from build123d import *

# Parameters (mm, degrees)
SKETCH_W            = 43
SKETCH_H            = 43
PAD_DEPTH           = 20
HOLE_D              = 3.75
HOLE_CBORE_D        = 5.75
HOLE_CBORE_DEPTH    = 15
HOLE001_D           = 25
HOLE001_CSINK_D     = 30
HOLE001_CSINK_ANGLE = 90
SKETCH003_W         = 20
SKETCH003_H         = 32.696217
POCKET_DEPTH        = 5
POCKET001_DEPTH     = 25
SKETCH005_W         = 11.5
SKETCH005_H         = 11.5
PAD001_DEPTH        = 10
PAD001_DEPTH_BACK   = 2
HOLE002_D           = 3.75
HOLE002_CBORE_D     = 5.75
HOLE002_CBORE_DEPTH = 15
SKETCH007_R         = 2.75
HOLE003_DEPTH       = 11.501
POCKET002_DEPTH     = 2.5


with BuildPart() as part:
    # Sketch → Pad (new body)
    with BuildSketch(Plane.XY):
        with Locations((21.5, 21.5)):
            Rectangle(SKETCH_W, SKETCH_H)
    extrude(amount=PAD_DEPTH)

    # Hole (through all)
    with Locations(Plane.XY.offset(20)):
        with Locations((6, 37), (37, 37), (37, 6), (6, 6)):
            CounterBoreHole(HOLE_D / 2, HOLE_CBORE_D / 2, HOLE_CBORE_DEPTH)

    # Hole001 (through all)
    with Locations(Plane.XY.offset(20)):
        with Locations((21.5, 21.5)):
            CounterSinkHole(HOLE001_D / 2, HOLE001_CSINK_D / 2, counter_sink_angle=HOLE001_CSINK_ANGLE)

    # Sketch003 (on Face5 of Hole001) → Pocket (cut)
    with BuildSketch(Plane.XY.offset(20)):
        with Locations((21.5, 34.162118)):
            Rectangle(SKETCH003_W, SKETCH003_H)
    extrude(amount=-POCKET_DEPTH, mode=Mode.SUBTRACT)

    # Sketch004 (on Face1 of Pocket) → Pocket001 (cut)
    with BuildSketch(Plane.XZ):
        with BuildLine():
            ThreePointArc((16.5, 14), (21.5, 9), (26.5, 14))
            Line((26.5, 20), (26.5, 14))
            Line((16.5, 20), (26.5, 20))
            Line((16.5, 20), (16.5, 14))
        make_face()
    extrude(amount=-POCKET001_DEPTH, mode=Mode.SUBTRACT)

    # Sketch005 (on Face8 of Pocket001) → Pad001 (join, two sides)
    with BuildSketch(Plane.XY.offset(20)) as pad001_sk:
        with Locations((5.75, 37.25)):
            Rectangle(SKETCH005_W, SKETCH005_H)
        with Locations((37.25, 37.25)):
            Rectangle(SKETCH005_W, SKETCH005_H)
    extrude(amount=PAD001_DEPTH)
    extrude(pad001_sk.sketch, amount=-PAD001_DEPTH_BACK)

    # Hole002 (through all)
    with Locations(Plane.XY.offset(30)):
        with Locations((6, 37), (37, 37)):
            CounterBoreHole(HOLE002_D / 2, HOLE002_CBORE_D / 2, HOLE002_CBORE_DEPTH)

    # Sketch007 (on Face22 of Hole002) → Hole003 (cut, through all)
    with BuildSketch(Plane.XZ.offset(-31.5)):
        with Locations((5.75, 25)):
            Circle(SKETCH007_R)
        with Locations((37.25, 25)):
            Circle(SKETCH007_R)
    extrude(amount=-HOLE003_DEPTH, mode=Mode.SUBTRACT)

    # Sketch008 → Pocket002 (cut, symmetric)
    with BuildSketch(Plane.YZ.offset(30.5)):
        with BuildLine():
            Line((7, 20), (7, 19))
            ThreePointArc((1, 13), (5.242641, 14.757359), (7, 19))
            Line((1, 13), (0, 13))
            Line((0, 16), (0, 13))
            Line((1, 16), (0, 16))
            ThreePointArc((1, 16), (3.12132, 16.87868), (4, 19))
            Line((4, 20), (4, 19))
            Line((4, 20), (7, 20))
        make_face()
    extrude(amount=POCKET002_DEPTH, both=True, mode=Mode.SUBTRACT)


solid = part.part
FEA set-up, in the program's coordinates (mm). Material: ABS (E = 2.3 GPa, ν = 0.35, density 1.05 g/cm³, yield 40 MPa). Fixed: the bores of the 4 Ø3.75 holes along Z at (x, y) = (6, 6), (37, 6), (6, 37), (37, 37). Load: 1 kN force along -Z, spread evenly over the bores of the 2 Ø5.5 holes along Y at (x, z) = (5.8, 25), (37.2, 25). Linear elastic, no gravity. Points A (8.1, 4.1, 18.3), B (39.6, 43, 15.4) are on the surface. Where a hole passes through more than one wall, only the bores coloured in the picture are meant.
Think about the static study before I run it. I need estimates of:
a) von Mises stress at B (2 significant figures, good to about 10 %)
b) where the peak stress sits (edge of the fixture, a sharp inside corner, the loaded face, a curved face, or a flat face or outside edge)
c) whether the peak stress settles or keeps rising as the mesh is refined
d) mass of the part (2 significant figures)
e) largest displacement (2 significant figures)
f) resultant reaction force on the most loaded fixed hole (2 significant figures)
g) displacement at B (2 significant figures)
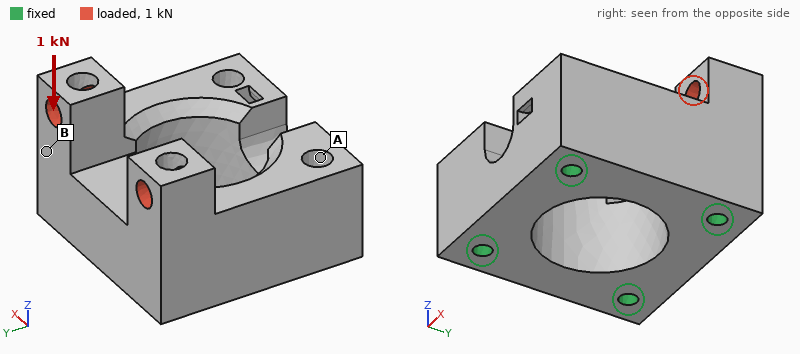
5.2 MPa
edge of the fixture
keeps rising
26 g
0.12 mm
500 N
0.056 mm
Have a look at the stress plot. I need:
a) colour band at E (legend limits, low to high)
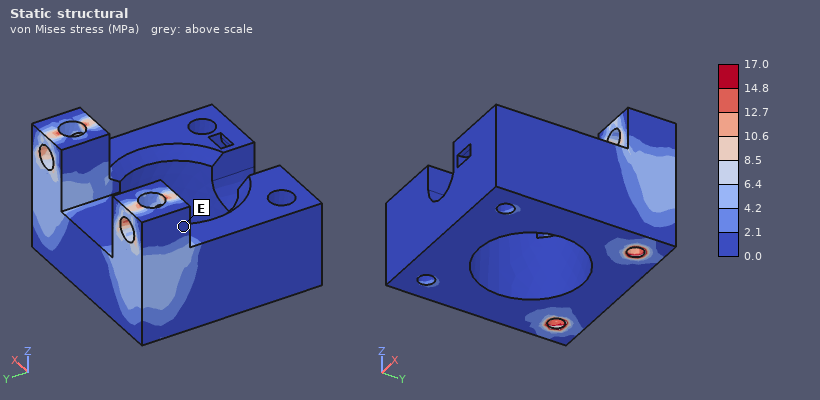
0.0 to 2.1 MPa
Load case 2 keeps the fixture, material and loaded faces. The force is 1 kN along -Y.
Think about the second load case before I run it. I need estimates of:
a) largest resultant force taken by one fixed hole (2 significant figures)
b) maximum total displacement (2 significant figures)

490 N
0.34 mm
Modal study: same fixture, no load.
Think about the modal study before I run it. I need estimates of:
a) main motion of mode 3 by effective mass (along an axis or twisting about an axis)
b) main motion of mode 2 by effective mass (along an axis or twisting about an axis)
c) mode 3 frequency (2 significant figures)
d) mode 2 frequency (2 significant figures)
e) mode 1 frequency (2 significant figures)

along Y
along X
5500 Hz
4600 Hz
4200 Hz
